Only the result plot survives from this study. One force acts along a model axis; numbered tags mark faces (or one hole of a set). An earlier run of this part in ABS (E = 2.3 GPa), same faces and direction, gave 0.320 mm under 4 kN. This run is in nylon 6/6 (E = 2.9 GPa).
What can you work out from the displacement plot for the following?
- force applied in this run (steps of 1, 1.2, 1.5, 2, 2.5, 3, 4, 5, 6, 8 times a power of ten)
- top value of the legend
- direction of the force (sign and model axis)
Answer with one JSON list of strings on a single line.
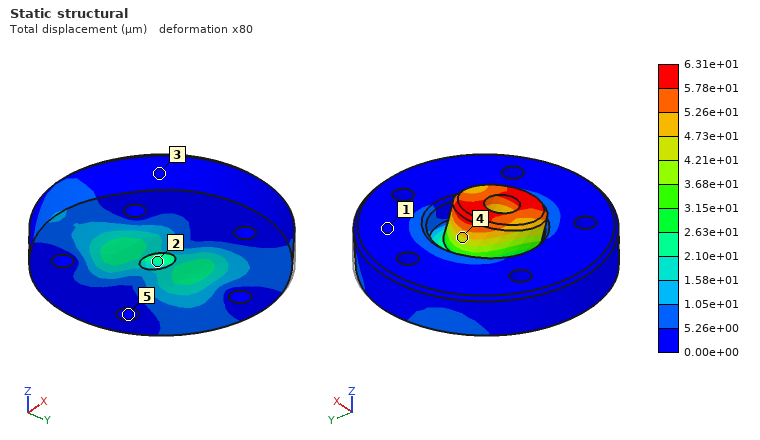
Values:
["1 kN", "6.31e+01 µm", "-Y"]
